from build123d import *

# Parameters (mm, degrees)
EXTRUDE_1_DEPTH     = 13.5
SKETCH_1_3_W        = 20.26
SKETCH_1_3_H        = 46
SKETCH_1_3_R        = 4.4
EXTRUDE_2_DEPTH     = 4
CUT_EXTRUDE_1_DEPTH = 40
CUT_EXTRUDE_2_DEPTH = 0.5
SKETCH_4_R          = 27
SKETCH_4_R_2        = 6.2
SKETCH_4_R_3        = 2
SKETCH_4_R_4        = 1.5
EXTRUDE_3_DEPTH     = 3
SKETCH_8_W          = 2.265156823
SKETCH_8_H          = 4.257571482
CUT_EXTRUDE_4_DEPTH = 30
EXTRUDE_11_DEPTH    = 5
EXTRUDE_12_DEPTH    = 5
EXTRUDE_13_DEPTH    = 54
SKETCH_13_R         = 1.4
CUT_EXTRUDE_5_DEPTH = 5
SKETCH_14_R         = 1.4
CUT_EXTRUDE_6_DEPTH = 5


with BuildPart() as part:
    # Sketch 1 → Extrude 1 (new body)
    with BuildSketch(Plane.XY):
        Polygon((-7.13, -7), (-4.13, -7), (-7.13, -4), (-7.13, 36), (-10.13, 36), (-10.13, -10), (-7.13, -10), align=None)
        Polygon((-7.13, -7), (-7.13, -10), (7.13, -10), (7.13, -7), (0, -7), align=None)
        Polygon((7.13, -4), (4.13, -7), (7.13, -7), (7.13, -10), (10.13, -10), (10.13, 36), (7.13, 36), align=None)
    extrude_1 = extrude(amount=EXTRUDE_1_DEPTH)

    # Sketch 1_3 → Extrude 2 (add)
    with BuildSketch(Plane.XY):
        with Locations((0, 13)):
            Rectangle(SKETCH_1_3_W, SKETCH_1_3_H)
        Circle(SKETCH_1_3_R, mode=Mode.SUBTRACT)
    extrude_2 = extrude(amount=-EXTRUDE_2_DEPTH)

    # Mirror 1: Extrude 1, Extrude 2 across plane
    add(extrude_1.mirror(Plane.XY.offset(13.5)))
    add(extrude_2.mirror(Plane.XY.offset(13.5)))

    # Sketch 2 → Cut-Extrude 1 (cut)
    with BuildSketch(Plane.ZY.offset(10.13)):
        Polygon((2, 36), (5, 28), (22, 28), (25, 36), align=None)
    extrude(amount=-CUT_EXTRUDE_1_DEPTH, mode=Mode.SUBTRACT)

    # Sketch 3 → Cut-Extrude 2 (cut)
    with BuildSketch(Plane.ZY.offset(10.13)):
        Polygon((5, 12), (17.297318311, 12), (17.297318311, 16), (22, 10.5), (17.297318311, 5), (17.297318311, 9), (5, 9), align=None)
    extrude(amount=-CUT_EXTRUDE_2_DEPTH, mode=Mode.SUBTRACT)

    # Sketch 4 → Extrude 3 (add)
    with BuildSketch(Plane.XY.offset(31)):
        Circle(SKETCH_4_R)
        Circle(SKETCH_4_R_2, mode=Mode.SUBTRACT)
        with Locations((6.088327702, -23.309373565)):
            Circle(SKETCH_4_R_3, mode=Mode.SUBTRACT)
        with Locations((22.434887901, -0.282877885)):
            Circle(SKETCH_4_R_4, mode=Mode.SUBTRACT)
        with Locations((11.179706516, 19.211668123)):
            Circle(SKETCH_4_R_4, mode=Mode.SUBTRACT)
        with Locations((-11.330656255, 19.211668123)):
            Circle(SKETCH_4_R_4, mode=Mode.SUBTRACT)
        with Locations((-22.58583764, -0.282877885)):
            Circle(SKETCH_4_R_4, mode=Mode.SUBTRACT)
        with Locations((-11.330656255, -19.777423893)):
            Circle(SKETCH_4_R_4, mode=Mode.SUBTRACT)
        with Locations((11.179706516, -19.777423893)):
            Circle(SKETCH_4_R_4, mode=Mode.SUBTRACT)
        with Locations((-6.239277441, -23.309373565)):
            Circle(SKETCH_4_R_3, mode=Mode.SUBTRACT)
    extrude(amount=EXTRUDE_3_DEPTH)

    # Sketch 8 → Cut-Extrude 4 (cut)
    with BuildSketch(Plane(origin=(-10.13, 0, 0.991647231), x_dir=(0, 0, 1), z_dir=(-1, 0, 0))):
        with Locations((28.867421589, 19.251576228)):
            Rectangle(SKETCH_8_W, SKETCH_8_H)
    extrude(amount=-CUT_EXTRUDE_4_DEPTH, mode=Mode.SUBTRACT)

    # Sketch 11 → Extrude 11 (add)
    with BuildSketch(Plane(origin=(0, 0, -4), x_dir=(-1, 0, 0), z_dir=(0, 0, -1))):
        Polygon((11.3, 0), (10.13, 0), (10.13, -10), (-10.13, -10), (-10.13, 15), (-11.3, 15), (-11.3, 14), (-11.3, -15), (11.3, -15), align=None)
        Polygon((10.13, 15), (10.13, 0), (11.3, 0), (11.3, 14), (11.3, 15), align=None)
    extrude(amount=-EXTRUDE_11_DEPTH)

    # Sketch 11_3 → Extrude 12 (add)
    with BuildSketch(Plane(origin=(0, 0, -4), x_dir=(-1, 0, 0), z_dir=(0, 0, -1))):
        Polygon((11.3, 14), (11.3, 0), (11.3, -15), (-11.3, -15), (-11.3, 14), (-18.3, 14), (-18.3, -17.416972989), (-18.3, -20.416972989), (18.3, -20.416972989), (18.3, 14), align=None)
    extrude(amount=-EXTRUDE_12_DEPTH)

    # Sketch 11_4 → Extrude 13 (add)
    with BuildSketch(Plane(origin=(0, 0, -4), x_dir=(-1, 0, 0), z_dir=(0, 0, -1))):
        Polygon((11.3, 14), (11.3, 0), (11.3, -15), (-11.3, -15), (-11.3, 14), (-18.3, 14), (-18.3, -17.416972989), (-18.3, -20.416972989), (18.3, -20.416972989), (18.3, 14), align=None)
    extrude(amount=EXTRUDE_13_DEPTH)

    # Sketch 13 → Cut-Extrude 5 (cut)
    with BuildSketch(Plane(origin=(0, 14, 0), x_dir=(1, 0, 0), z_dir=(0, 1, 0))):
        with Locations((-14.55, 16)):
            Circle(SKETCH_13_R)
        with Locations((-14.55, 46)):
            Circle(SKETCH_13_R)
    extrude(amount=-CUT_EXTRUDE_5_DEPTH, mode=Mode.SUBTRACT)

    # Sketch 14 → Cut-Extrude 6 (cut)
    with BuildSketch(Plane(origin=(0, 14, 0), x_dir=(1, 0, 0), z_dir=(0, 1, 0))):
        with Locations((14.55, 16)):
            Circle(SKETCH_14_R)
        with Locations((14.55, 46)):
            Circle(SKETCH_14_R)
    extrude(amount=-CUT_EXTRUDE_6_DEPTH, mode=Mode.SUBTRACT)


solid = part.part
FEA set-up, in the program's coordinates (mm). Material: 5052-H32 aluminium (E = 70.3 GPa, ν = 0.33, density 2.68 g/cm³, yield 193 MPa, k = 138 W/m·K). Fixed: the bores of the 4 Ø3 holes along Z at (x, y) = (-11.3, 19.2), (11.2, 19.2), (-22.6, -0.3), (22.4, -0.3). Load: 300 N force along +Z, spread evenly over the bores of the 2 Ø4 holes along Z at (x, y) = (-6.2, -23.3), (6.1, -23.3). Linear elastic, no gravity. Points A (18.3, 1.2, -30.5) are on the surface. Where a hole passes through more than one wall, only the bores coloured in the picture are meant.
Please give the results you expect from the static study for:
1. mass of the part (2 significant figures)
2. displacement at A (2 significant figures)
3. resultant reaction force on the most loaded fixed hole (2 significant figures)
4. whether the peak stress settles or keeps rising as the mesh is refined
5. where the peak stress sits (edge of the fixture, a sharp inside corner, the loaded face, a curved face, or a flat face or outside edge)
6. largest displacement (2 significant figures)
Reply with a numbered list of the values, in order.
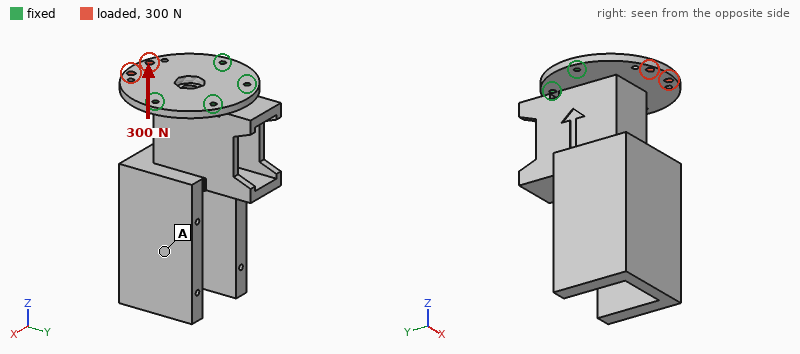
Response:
1. 150 g
2. 0.075 mm
3. 280 N
4. keeps rising
5. edge of the fixture
6. 0.15 mm
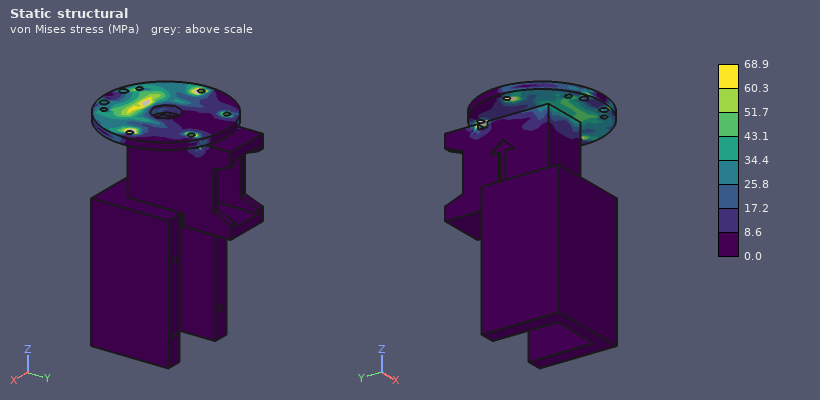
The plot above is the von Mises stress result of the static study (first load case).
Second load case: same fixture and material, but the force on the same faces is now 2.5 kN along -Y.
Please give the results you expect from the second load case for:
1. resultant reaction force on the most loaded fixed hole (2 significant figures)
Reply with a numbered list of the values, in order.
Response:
1. 740 N
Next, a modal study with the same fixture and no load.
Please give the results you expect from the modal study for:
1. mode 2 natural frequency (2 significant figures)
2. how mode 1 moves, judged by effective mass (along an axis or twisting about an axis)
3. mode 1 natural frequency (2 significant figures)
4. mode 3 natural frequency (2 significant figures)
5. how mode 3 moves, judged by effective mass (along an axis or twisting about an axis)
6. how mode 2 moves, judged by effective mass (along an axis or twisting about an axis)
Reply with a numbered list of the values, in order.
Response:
1. 810 Hz
2. along Y
3. 730 Hz
4. 2600 Hz
5. twisting about Z
6. along X
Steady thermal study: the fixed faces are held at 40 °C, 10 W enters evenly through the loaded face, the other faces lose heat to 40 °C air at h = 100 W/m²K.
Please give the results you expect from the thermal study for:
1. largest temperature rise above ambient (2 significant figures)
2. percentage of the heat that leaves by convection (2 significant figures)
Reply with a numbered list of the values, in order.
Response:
1. 18 K
2. 37 %
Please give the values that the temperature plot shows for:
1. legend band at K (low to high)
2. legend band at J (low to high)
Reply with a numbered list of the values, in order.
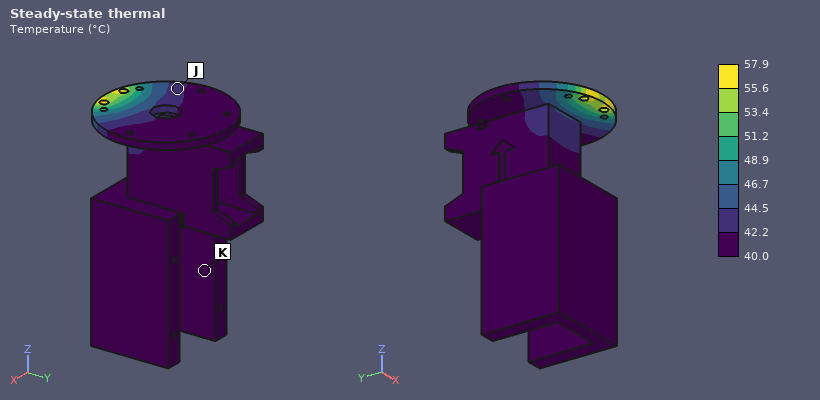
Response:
1. 40.0 to 42.2 °C
2. 42.2 to 44.5 °C
